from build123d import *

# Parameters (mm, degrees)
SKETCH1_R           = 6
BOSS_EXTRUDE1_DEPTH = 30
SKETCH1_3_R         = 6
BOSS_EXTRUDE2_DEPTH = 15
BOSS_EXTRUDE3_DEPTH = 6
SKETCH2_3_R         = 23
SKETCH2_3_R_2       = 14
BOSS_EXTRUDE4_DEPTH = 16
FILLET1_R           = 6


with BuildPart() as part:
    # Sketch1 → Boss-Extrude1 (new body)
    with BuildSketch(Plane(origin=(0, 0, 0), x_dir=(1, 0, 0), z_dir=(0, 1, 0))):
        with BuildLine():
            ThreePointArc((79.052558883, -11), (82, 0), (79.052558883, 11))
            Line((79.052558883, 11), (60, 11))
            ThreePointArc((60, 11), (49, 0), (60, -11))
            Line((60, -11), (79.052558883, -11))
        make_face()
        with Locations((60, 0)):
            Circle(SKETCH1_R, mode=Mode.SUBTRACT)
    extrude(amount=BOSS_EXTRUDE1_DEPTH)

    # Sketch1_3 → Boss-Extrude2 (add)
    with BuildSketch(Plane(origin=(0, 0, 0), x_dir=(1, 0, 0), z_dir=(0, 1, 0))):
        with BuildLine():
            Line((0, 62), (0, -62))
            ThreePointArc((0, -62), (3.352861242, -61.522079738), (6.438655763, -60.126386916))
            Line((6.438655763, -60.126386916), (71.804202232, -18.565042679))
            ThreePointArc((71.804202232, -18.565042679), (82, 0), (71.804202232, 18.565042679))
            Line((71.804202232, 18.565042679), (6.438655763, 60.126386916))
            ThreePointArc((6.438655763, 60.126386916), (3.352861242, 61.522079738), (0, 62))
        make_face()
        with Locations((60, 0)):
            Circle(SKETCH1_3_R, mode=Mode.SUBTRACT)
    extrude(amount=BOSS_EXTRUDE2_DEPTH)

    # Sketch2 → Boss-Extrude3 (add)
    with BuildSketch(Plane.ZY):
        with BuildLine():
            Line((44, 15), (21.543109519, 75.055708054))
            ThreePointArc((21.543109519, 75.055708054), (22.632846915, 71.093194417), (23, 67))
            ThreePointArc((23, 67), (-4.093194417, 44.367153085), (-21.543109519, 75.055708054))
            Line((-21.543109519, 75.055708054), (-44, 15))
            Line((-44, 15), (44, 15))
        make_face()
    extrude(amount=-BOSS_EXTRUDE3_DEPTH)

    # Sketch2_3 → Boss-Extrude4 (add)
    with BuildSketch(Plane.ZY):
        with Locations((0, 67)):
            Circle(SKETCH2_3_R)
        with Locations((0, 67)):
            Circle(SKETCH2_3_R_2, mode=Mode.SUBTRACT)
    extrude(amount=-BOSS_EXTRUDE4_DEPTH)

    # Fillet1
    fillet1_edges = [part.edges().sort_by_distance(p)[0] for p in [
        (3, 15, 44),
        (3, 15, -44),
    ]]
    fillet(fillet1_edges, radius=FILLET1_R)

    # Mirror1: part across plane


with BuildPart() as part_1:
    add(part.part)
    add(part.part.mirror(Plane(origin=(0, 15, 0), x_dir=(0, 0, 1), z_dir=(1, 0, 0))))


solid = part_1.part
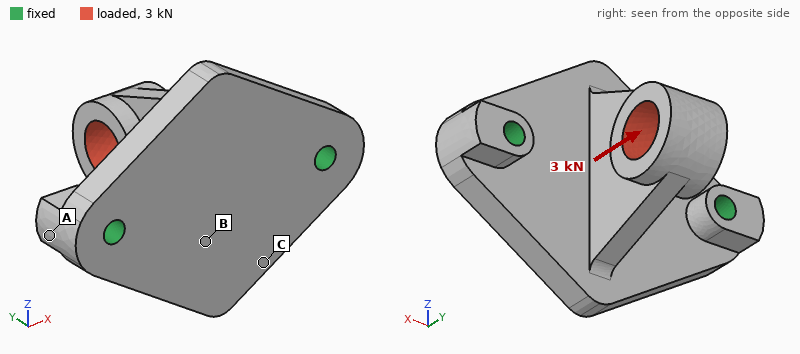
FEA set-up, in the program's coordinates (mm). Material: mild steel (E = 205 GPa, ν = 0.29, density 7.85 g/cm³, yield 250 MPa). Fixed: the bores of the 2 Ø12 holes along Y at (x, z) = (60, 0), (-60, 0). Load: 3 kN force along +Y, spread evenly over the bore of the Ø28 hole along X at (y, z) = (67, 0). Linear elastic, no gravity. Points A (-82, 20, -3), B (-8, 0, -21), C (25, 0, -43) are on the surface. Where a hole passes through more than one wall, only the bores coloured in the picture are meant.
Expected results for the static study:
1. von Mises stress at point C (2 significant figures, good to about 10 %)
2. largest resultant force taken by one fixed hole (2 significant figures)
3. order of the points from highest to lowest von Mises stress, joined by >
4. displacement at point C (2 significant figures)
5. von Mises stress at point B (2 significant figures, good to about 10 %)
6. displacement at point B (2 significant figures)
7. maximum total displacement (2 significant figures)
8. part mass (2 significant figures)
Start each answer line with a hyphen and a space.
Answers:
- 5.1 MPa
- 1.5 kN
- B > C > A
- 5.5 µm
- 9.3 MPa
- 6.3 µm
- 8.2 µm
- 2.1 kg
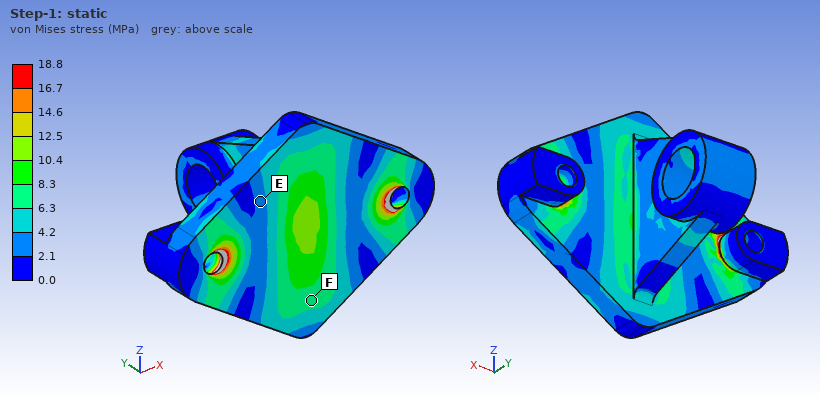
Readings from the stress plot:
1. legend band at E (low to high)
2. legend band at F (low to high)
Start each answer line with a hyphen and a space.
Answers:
- 2.1 to 4.2 MPa
- 6.3 to 8.3 MPa
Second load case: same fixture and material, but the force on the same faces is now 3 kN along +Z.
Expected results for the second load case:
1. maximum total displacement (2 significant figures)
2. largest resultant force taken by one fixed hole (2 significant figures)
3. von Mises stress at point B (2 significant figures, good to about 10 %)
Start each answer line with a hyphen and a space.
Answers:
- 57 µm
- 1.5 kN
- 12 MPa
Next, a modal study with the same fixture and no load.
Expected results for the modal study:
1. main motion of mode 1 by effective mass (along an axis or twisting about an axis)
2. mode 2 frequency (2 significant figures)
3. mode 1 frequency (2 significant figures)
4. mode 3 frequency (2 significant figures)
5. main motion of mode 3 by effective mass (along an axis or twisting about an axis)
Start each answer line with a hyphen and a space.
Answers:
- along X
- 1800 Hz
- 1600 Hz
- 3000 Hz
- along Y
